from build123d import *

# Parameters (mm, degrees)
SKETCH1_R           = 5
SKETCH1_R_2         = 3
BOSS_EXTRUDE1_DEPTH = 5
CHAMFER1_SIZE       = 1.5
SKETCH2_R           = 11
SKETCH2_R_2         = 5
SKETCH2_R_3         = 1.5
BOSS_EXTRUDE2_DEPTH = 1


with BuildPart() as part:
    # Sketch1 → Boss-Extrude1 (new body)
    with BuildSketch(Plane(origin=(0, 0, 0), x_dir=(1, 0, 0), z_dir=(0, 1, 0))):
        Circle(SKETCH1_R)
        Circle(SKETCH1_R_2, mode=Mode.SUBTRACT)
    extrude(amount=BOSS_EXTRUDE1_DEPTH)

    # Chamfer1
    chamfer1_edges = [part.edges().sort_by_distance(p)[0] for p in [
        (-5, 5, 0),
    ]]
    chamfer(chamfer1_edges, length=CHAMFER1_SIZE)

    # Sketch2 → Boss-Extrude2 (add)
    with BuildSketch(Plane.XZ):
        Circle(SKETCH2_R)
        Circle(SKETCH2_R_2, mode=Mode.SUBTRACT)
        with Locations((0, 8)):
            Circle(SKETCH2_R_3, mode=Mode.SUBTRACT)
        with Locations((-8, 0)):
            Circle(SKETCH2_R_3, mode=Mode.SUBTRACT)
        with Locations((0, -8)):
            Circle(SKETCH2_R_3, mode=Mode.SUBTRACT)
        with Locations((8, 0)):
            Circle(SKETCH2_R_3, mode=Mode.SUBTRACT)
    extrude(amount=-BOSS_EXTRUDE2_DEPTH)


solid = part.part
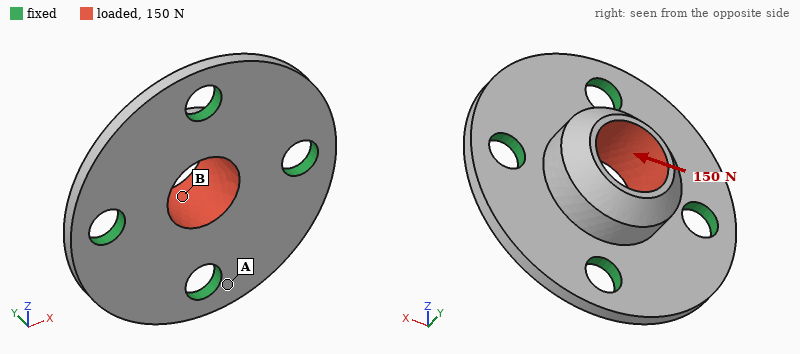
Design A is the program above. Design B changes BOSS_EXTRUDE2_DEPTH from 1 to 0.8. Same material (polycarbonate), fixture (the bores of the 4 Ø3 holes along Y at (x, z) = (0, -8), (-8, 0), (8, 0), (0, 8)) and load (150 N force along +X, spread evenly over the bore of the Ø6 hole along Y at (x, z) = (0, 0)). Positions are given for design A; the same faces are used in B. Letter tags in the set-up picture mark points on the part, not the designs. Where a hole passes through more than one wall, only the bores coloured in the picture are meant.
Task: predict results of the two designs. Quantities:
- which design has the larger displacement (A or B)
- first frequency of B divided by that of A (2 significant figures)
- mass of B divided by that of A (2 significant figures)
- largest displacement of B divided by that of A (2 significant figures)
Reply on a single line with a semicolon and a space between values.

B; 0.82; 0.89; 1.4
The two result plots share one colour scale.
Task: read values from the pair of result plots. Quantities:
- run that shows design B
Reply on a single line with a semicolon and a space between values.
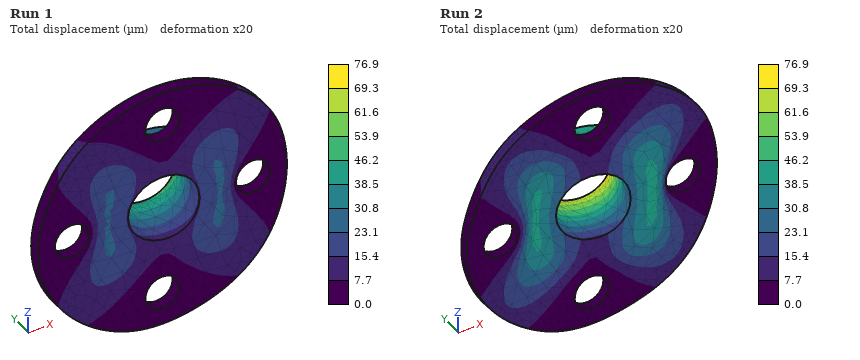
Run 2
